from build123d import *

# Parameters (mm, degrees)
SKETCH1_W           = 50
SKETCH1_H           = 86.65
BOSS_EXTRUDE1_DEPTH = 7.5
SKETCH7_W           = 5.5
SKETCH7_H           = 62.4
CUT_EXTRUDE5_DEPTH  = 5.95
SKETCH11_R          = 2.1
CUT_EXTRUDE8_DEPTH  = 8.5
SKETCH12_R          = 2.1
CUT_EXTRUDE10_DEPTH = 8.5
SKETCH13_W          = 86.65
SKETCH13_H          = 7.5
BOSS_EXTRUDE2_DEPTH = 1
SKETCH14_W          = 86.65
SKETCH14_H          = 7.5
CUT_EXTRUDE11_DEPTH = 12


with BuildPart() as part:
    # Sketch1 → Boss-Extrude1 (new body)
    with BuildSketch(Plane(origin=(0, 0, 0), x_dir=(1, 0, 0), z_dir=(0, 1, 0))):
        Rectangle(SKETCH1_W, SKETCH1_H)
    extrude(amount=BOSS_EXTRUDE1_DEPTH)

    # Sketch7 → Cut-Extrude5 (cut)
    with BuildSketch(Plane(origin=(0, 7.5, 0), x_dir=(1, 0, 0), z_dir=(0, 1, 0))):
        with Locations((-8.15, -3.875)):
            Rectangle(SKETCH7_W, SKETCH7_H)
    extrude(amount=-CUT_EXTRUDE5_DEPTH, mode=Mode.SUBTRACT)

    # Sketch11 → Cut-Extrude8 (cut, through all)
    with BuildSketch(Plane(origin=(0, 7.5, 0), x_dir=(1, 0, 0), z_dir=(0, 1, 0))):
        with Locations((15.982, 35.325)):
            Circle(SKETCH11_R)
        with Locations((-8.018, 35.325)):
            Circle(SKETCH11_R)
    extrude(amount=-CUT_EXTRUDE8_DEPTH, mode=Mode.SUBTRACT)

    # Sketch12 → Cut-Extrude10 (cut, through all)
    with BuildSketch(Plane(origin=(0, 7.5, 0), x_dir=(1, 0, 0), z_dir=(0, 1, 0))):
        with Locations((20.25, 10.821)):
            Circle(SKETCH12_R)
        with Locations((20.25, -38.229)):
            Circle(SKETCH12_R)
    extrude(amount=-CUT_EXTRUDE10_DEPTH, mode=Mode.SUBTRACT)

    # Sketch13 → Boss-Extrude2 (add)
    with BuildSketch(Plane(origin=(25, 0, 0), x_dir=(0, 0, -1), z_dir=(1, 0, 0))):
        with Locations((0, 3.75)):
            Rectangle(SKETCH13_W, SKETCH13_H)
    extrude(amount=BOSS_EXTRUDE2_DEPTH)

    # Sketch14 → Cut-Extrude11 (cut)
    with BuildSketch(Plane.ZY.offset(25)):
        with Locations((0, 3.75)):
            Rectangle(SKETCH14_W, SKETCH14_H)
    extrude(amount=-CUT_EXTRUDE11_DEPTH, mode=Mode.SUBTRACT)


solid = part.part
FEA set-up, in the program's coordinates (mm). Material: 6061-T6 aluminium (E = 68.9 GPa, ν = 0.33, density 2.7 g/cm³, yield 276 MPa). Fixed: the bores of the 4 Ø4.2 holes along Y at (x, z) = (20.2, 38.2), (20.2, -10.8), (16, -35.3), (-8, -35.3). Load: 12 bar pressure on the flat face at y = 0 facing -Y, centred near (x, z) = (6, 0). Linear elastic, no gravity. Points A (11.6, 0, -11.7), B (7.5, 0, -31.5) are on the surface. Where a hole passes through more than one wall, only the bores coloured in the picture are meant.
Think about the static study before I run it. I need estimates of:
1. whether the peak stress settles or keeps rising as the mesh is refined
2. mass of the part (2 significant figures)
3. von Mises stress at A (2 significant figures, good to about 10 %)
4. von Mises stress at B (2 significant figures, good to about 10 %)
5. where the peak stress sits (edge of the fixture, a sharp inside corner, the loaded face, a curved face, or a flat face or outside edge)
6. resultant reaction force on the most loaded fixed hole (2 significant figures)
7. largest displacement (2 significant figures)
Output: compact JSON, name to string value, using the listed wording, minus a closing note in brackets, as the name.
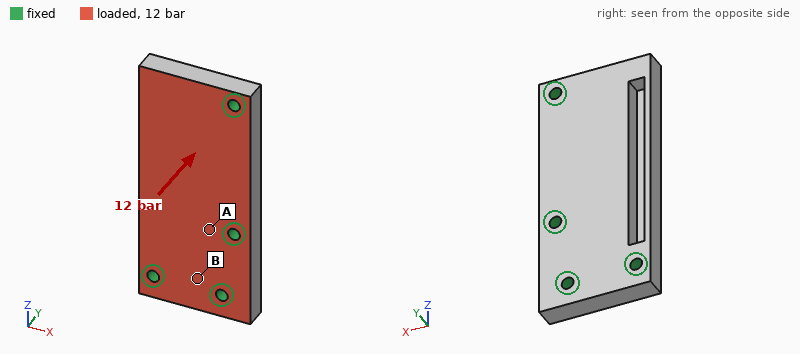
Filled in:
{"whether the peak stress settles or keeps rising as the mesh is refined": "keeps rising", "mass of the part": "62 g", "von Mises stress at A": "35 MPa", "von Mises stress at B": "18 MPa", "where the peak stress sits": "edge of the fixture", "resultant reaction force on the most loaded fixed hole": "1.4 kN", "largest displacement": "0.13 mm"}
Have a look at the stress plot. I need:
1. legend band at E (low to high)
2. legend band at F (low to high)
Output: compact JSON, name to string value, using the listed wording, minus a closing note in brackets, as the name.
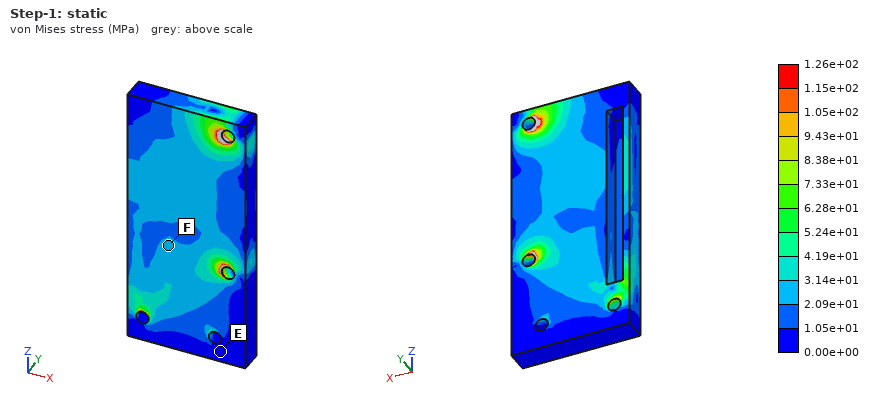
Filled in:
{"legend band at E": "0.00e+00 to 1.05e+01 MPa", "legend band at F": "2.09e+01 to 3.14e+01 MPa"}
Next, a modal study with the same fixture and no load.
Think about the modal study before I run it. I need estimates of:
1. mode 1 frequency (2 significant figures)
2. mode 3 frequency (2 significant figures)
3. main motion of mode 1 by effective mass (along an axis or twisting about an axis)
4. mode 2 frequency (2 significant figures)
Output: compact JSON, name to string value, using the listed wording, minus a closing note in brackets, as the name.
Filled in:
{"mode 1 frequency": "5300 Hz", "mode 3 frequency": "12 kHz", "main motion of mode 1 by effective mass": "along Y", "mode 2 frequency": "10 kHz"}
